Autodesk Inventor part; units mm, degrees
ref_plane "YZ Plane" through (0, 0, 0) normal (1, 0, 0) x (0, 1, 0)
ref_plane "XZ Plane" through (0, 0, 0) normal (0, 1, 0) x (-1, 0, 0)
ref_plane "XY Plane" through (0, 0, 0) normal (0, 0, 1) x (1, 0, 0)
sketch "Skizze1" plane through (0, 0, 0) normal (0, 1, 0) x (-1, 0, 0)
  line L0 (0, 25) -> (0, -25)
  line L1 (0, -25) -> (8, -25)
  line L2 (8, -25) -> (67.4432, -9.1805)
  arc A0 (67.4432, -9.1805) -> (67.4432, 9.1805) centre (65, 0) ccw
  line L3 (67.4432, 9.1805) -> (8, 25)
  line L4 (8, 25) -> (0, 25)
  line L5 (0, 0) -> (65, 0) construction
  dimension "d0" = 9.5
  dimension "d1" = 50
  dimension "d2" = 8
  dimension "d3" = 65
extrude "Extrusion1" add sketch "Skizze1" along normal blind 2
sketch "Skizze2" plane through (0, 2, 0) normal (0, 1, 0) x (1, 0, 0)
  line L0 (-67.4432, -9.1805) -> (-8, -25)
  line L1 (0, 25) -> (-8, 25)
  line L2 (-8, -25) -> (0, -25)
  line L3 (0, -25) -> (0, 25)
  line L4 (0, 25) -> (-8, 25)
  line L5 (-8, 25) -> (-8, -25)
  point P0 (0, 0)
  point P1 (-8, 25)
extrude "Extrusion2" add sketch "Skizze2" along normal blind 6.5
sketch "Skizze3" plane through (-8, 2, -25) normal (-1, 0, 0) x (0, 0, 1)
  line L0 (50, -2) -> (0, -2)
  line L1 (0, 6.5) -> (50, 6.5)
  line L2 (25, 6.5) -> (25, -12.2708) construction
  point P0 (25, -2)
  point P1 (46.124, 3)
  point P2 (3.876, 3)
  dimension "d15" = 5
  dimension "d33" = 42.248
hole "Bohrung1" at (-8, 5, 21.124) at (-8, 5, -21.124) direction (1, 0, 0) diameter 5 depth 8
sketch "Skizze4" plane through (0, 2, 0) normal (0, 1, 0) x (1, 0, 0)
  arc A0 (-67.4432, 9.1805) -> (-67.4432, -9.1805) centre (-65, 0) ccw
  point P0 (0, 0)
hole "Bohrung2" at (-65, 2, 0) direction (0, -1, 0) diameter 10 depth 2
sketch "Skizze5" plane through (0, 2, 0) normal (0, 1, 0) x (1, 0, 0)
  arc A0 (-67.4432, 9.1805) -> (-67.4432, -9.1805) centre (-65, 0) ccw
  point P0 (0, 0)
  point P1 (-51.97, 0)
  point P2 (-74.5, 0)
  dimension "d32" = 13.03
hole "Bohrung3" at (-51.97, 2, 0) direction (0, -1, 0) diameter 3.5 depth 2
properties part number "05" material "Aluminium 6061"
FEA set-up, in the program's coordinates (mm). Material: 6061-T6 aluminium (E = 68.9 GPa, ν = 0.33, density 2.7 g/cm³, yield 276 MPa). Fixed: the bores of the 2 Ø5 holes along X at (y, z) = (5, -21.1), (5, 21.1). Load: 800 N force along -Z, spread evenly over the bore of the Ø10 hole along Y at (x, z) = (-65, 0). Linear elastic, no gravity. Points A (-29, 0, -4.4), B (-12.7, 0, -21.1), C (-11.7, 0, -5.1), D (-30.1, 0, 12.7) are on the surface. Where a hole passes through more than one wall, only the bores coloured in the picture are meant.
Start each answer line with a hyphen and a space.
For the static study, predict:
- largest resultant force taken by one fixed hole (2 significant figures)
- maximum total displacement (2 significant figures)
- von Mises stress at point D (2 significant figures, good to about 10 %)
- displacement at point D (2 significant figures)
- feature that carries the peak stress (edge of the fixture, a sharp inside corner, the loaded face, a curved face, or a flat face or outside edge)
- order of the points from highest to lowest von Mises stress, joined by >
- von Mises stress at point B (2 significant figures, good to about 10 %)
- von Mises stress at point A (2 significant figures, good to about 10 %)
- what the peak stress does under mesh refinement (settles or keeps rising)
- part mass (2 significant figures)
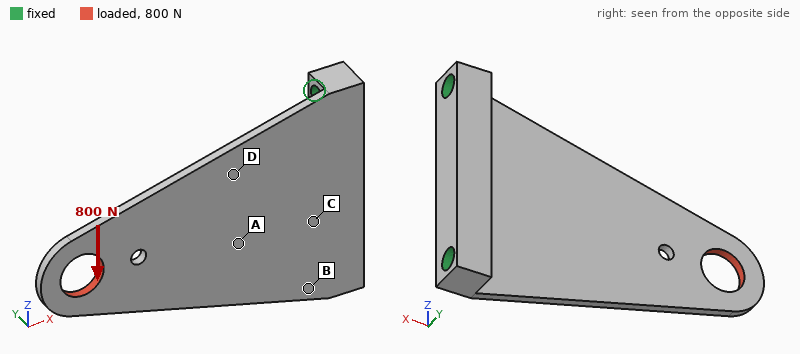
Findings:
- 1.3 kN
- 0.14 mm
- 41 MPa
- 0.025 mm
- edge of the fixture
- B > D > A > C
- 52 MPa
- 18 MPa
- keeps rising
- 19 g
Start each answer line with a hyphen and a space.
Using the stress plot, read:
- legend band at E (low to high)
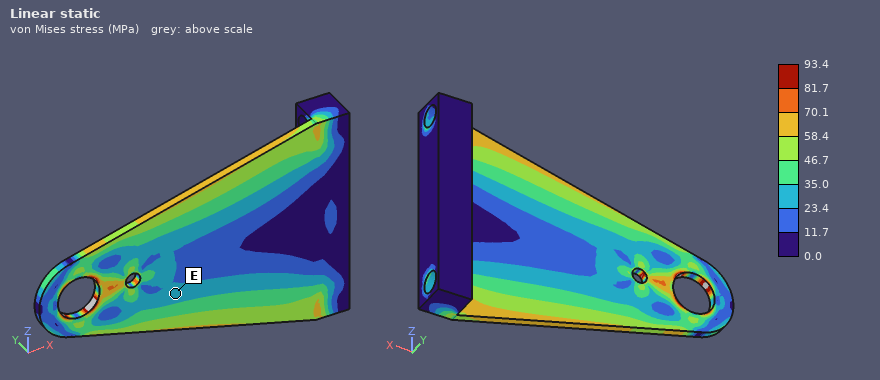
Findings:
- 23.4 to 35.0 MPa
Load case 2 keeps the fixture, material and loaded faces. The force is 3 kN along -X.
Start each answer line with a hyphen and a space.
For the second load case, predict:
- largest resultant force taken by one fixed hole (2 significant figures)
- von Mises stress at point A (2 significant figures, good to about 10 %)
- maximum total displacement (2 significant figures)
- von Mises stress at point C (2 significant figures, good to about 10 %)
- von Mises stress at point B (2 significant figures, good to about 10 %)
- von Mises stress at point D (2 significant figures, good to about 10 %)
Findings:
- 1.6 kN
- 36 MPa
- 0.12 mm
- 19 MPa
- 52 MPa
- 42 MPa
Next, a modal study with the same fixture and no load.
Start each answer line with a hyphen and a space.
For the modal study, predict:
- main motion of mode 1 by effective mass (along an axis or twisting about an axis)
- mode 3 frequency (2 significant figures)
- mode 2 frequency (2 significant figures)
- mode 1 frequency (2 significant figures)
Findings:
- along Y
- 2600 Hz
- 2500 Hz
- 570 Hz
